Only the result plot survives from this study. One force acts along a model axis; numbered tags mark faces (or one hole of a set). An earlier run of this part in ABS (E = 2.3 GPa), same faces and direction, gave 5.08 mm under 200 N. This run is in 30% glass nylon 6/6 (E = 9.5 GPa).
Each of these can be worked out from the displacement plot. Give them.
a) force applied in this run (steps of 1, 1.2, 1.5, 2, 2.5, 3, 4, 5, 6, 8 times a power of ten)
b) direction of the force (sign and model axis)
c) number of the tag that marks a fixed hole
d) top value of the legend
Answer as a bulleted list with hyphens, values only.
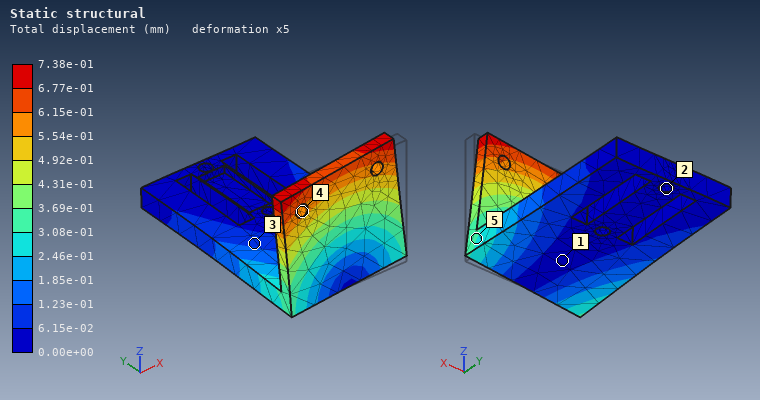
- 120 N
- -X
- 2
- 7.38e-01 mm
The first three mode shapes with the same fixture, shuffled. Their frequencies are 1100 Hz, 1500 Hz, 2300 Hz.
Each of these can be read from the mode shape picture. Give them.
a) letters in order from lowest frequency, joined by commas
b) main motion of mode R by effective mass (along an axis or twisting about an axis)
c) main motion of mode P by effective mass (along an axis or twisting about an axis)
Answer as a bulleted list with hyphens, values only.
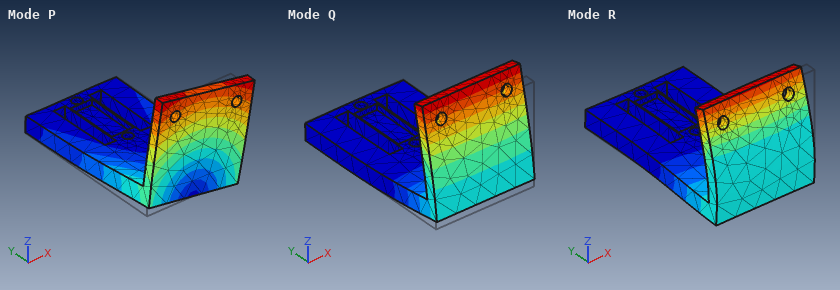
- Q, P, R
- along Z
- along X
